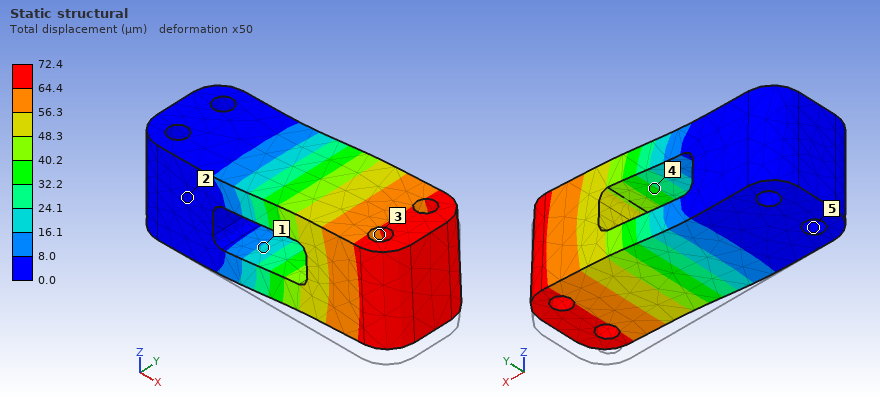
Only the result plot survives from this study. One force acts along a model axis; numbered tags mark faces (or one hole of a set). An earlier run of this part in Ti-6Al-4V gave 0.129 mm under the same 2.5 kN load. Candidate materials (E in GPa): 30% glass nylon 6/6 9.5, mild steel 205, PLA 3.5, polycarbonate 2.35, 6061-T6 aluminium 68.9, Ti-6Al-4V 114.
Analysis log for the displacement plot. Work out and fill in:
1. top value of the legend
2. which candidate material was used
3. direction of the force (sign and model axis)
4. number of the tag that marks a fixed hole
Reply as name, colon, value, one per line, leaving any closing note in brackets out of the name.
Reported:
top value of the legend: 72.4 µm
which candidate material was used: mild steel
direction of the force: +Z
number of the tag that marks a fixed hole: 5
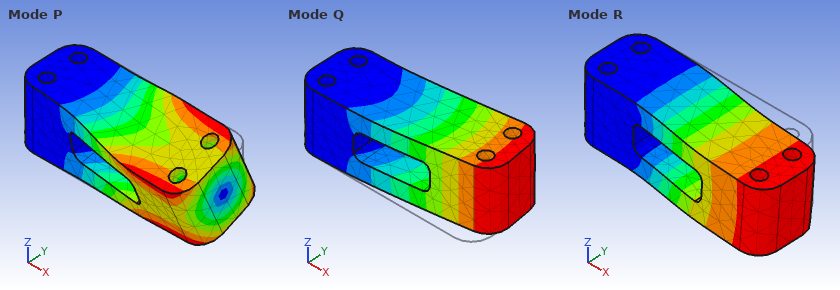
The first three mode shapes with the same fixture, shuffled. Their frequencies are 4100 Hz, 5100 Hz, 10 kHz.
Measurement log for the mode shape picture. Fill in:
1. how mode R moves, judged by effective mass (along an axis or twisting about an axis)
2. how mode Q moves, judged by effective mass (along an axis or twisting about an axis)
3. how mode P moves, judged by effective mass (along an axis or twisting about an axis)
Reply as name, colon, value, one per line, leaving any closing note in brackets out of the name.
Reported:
how mode R moves, judged by effective mass: along Z
how mode Q moves, judged by effective mass: along Y
how mode P moves, judged by effective mass: twisting about X
